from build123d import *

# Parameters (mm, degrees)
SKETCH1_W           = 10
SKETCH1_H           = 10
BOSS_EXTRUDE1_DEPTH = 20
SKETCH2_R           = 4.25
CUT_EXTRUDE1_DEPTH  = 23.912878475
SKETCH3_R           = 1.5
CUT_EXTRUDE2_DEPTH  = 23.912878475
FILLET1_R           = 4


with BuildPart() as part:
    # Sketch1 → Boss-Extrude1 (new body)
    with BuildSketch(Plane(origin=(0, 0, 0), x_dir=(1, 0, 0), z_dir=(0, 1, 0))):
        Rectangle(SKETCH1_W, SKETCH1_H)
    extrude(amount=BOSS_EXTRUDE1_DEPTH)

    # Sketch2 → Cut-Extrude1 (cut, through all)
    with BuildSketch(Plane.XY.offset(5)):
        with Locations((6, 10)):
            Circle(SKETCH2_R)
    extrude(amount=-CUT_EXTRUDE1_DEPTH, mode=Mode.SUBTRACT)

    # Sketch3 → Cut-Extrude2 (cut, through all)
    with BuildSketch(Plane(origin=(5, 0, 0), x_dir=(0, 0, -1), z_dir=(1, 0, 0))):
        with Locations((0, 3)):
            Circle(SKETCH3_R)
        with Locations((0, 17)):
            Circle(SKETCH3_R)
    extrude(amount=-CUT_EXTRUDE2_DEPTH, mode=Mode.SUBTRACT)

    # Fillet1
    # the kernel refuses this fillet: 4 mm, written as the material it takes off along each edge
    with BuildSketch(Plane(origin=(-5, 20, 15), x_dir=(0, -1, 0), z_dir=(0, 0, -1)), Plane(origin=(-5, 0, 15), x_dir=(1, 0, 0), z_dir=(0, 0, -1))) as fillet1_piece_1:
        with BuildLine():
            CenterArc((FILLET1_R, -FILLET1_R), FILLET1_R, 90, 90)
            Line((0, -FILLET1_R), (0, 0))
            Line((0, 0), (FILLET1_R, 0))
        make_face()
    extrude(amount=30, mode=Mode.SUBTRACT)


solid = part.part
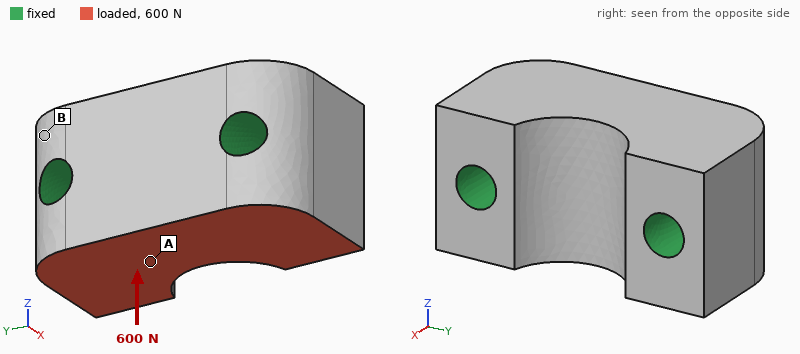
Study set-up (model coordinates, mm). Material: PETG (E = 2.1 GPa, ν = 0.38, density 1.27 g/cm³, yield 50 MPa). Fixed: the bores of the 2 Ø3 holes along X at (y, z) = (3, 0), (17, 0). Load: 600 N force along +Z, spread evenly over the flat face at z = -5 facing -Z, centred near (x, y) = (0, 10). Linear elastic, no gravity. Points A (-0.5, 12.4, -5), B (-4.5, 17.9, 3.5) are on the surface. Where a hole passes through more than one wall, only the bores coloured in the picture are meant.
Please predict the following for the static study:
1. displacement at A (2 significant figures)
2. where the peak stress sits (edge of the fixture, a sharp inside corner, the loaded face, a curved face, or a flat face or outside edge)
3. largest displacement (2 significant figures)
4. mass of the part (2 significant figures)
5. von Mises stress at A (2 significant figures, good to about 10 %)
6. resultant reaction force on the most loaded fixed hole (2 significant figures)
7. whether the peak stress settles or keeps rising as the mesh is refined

14 µm
edge of the fixture
21 µm
2.0 g
3.0 MPa
300 N
keeps rising
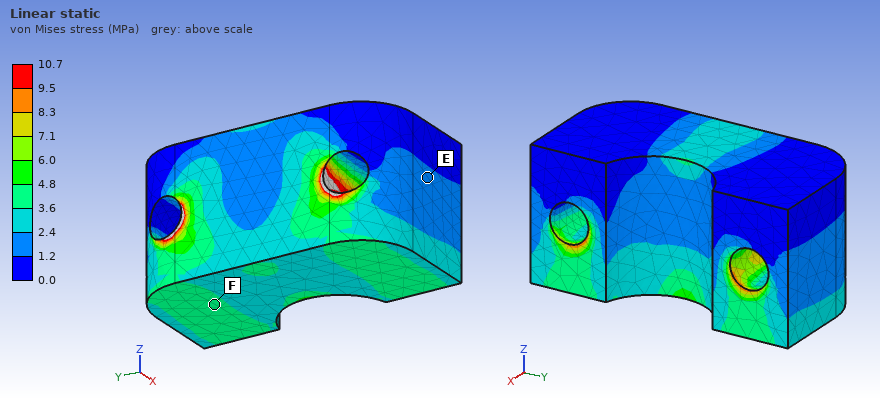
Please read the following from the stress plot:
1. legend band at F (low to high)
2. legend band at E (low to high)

3.6 to 4.8 MPa
1.2 to 2.4 MPa
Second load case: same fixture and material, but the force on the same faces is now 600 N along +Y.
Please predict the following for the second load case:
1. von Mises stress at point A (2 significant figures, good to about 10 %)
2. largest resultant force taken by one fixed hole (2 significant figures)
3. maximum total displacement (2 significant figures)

6.4 MPa
330 N
44 µm
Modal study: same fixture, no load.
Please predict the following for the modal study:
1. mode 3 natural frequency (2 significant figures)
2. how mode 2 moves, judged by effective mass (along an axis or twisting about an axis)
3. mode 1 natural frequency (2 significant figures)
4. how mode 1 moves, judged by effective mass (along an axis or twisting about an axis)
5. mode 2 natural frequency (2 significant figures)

29 kHz
along X
24 kHz
along Z
26 kHz
